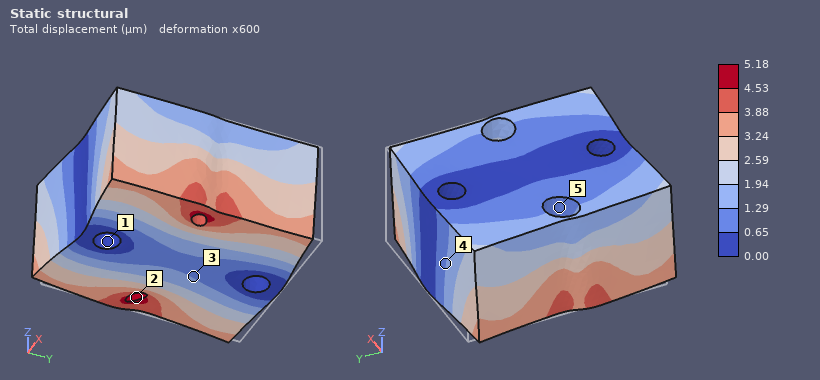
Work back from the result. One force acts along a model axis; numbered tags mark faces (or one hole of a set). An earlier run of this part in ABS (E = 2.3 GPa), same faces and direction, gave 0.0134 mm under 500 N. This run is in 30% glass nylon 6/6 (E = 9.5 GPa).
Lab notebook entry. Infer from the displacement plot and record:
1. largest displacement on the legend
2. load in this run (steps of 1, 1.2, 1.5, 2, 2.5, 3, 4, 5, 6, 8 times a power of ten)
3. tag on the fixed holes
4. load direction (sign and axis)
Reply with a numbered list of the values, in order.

1. 5.18 µm
2. 800 N
3. 1
4. -Y
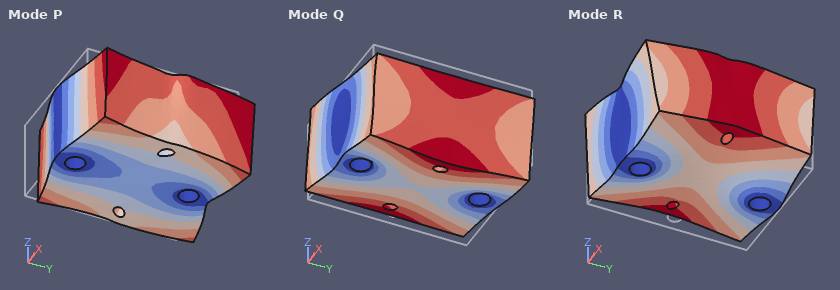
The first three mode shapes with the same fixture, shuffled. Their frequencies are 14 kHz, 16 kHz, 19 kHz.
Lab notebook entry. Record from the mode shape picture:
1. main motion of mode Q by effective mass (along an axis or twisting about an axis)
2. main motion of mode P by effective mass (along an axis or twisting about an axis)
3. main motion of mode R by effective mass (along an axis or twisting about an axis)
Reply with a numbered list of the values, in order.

1. twisting about Y
2. along Y
3. along Z
